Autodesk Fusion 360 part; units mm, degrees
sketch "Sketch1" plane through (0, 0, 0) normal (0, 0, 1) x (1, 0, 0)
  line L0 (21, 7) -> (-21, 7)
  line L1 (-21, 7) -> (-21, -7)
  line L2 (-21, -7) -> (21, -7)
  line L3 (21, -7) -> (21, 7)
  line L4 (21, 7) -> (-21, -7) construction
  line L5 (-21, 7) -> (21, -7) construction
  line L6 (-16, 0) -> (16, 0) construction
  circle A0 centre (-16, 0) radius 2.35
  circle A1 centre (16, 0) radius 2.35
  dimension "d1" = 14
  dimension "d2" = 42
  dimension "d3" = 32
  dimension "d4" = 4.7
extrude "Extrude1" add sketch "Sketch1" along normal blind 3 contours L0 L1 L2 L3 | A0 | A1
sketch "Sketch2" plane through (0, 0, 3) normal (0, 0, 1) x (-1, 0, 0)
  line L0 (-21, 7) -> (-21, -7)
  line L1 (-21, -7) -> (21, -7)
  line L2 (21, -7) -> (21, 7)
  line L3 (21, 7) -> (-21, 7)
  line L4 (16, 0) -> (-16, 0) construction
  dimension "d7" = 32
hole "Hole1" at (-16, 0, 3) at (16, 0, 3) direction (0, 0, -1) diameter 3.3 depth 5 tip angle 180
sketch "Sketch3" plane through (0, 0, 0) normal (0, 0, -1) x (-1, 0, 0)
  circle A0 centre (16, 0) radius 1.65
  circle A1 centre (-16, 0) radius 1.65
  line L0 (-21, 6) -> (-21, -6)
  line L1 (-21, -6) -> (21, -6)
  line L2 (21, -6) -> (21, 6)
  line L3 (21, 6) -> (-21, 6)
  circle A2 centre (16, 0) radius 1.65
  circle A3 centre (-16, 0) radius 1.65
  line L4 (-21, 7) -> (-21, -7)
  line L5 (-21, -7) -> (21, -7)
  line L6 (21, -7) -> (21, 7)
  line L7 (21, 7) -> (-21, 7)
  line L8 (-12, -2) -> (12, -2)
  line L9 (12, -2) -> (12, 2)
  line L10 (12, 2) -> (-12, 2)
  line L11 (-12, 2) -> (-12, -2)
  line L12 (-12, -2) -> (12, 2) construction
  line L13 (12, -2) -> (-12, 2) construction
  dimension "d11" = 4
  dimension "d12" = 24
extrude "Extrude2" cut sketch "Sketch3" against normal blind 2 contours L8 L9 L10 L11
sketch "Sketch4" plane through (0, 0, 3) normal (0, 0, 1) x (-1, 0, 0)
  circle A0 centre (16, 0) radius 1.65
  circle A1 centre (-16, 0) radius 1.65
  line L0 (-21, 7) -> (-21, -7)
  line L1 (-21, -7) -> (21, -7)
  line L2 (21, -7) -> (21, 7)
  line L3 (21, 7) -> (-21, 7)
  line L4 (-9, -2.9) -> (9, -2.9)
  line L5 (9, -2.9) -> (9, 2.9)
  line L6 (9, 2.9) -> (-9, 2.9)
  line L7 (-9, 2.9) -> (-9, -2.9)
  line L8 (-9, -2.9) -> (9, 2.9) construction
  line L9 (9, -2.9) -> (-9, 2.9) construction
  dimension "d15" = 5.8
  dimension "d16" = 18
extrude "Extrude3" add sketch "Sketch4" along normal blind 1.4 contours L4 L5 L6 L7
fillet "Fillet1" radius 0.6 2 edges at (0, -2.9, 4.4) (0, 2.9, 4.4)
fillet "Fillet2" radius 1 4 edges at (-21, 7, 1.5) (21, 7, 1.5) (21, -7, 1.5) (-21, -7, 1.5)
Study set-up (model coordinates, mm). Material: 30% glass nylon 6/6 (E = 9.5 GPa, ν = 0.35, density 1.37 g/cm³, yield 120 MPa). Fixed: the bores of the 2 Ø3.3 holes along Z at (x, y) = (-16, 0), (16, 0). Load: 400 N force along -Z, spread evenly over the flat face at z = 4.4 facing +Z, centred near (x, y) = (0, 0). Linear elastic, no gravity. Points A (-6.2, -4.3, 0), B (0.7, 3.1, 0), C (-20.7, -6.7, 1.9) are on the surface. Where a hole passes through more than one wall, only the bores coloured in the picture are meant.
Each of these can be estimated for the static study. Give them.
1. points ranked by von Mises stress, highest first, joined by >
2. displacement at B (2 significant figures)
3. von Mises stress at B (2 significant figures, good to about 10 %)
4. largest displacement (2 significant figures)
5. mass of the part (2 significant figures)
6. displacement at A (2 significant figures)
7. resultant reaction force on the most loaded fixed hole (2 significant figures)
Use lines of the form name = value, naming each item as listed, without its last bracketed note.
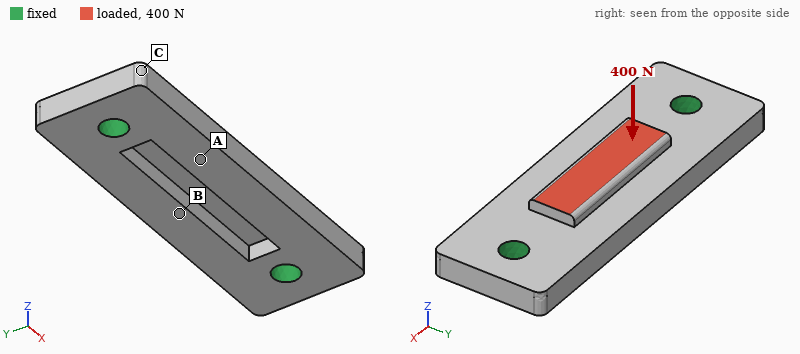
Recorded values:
points ranked by von Mises stress, highest first, joined by > = B > A > C
displacement at B = 0.16 mm
von Mises stress at B = 37 MPa
largest displacement = 0.17 mm
mass of the part = 2.3 g
displacement at A = 0.12 mm
resultant reaction force on the most loaded fixed hole = 220 N
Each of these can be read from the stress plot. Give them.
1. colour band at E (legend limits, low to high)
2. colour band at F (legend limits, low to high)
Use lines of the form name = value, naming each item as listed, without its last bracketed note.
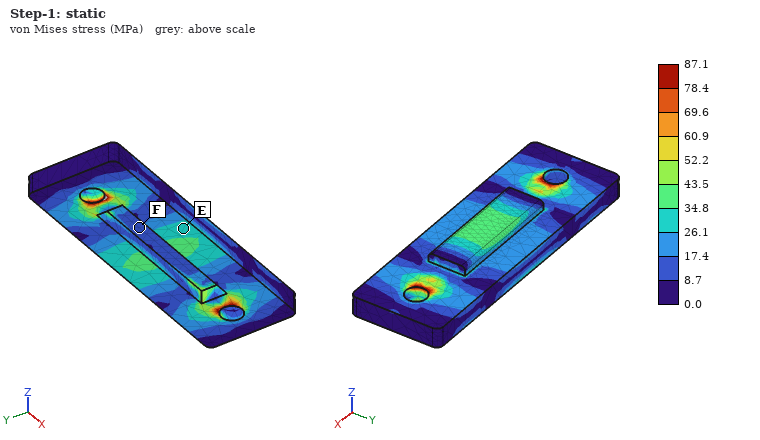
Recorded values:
colour band at E = 26.1 to 34.8 MPa
colour band at F = 8.7 to 17.4 MPa
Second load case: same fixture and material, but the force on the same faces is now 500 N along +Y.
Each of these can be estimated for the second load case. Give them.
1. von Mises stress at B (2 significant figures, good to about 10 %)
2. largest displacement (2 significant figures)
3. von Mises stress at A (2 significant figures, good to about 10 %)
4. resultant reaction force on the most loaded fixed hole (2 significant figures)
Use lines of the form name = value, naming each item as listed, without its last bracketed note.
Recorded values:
von Mises stress at B = 14 MPa
largest displacement = 0.13 mm
von Mises stress at A = 19 MPa
resultant reaction force on the most loaded fixed hole = 250 N
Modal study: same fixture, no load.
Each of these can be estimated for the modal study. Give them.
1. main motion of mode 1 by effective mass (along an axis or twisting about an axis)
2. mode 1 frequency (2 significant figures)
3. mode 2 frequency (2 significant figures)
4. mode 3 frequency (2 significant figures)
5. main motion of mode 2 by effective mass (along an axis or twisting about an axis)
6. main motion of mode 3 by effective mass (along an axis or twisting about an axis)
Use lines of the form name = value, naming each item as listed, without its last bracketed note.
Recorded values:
main motion of mode 1 by effective mass = along Z
mode 1 frequency = 8000 Hz
mode 2 frequency = 9700 Hz
mode 3 frequency = 15 kHz
main motion of mode 2 by effective mass = twisting about X
main motion of mode 3 by effective mass = along Y
